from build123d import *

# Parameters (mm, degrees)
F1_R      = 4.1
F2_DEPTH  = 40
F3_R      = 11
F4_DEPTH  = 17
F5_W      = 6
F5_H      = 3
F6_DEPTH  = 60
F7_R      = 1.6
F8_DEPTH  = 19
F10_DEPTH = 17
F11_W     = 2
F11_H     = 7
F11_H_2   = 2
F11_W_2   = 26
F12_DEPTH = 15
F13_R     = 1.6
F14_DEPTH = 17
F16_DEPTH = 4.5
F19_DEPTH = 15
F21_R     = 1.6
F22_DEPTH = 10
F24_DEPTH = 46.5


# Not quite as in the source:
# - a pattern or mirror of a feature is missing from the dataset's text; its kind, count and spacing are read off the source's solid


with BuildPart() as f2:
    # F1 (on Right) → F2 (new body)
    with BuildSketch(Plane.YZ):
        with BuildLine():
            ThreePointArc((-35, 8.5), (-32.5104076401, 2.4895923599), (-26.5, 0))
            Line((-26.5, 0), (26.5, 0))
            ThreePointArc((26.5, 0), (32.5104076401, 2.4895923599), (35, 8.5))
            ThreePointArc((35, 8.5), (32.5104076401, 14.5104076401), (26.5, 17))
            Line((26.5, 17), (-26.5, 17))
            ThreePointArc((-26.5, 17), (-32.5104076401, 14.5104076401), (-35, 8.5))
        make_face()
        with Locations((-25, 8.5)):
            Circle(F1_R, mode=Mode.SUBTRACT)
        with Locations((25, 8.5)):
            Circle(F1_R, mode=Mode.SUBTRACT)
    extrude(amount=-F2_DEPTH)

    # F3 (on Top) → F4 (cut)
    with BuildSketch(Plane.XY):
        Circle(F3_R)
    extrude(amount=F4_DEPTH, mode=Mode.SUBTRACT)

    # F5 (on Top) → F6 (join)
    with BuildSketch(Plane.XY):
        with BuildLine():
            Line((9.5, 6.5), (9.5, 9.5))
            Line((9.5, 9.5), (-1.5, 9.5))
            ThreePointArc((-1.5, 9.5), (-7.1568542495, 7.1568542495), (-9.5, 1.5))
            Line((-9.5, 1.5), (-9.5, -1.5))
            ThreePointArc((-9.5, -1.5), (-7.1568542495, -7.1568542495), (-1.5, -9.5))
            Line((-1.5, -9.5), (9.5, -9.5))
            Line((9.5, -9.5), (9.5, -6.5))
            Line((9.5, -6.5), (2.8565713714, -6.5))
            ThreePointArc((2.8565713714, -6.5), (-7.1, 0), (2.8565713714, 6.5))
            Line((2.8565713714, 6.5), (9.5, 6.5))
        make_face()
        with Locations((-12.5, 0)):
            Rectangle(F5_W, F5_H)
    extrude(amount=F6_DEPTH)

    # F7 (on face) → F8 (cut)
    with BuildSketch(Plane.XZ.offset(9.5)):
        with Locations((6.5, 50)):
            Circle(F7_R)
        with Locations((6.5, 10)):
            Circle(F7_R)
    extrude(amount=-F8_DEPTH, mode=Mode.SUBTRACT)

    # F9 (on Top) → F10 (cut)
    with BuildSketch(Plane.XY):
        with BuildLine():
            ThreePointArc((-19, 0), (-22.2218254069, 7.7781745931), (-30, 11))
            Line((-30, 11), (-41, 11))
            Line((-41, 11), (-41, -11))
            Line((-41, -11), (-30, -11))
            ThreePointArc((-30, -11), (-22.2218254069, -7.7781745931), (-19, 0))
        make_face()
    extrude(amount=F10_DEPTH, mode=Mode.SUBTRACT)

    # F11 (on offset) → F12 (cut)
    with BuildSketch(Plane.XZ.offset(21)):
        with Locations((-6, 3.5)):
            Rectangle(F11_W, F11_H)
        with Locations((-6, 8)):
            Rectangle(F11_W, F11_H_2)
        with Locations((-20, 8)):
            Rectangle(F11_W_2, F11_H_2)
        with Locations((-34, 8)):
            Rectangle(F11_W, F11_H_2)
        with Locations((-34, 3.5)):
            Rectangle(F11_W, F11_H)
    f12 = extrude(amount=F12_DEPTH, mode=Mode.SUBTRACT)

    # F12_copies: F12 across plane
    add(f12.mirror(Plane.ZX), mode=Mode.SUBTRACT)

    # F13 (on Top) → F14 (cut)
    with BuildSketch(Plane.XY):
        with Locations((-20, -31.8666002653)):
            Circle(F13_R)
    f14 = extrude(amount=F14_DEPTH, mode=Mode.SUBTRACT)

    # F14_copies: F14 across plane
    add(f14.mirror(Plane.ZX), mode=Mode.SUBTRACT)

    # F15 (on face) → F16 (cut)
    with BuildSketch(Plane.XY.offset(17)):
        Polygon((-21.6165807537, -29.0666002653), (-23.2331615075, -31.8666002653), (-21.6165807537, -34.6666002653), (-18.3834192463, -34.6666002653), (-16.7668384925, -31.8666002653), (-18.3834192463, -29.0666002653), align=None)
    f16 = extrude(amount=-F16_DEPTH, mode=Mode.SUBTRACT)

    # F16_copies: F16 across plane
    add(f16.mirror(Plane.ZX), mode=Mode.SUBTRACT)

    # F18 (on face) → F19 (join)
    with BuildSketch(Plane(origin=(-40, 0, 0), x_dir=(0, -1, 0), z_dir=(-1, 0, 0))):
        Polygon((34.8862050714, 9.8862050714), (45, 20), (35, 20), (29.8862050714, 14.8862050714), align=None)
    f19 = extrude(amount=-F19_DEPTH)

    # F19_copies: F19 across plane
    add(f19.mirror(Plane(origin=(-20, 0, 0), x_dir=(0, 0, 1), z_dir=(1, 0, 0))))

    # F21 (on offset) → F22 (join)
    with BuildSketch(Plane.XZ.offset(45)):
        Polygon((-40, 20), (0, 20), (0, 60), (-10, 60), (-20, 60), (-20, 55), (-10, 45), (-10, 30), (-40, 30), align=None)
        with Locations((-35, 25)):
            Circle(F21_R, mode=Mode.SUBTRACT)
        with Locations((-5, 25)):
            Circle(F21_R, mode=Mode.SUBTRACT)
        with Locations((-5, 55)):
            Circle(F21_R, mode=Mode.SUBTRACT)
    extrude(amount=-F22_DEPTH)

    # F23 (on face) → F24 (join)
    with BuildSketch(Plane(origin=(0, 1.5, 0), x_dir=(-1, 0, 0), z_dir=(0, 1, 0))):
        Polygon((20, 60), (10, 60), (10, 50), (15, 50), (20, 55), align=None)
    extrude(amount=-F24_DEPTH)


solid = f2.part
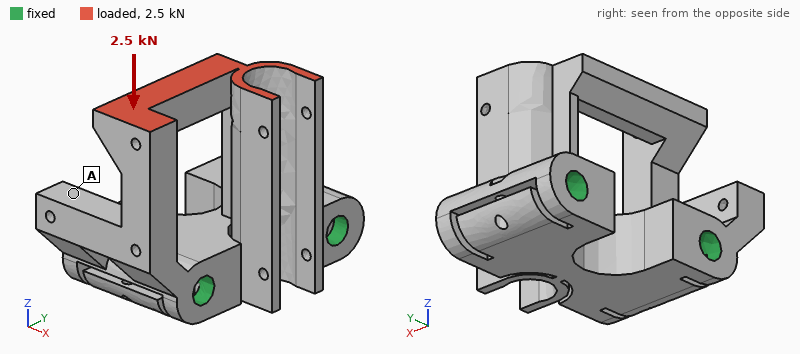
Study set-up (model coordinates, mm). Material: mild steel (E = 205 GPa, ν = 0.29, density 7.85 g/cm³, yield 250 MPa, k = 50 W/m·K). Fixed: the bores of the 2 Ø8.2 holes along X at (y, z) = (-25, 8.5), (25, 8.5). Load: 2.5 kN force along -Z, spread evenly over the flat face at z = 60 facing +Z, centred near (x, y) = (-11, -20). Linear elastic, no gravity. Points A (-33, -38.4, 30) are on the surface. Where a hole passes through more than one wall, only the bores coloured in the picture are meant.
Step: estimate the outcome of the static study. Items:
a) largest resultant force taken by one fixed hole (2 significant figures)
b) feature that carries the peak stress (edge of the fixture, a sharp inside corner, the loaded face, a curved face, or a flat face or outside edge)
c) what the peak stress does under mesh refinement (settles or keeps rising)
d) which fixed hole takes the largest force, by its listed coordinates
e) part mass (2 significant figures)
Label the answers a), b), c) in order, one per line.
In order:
a) 2.0 kN
b) a sharp inside corner
c) keeps rising
d) (-25, 8.5)
e) 400 g
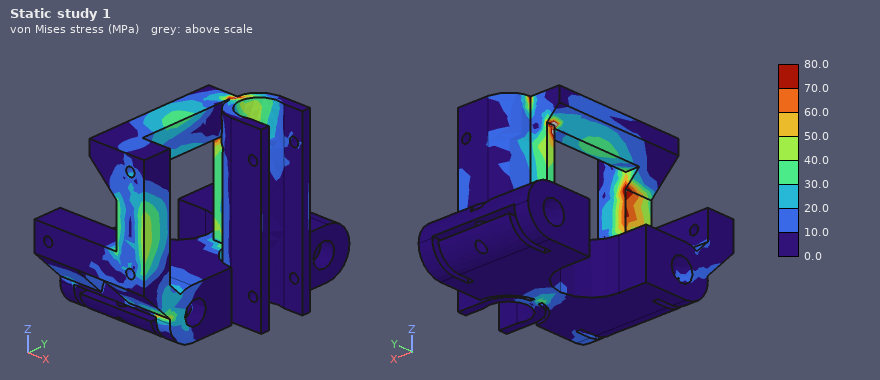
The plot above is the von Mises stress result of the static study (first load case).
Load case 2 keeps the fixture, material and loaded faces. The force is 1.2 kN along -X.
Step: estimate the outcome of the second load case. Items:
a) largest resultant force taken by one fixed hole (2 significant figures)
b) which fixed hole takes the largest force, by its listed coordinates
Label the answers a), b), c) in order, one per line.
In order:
a) 940 N
b) (-25, 8.5)
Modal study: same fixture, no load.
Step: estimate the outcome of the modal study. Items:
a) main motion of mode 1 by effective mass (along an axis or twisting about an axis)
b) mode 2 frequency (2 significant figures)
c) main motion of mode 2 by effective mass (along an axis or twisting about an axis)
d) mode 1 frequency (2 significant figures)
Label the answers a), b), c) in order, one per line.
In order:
a) along Y
b) 2500 Hz
c) along X
d) 2300 Hz
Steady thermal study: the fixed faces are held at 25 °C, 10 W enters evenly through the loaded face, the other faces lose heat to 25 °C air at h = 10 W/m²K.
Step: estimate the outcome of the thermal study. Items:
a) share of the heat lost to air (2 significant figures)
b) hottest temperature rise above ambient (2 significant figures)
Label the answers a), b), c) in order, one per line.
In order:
a) 22 %
b) 43 K
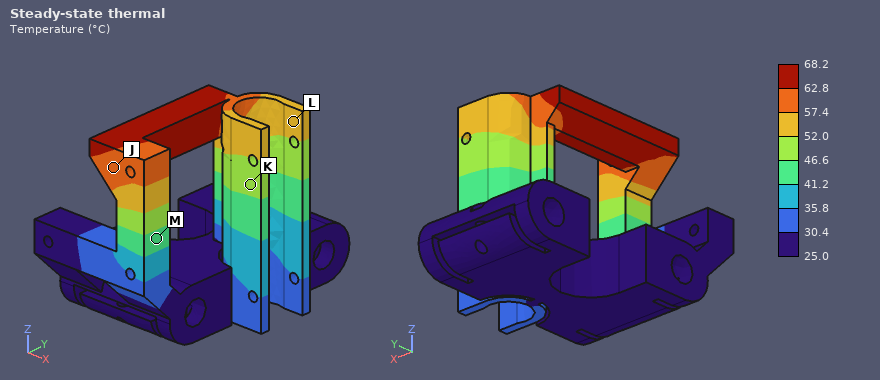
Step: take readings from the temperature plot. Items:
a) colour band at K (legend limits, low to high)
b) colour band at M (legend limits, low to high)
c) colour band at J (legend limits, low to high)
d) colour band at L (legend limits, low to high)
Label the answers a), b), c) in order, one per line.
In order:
a) 46.6 to 52.0 °C
b) 41.2 to 46.6 °C
c) 57.4 to 62.8 °C
d) 52.0 to 57.4 °C
